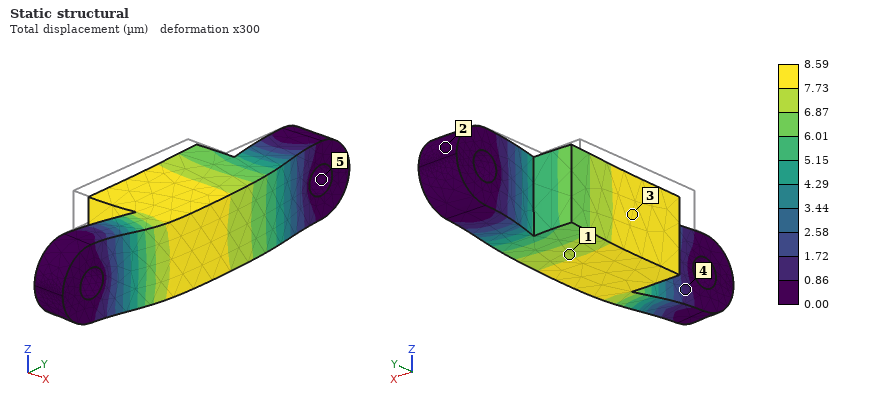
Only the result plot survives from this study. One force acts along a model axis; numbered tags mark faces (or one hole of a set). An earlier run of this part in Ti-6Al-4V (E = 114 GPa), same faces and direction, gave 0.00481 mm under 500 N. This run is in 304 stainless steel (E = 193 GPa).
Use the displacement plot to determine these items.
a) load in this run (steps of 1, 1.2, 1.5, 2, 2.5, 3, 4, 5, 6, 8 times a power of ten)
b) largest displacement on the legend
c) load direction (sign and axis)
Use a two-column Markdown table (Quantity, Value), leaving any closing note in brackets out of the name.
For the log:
| Quantity | Value |
|---|---|
| load in this run | 1.5 kN |
| largest displacement on the legend | 8.59 µm |
| load direction | +X |
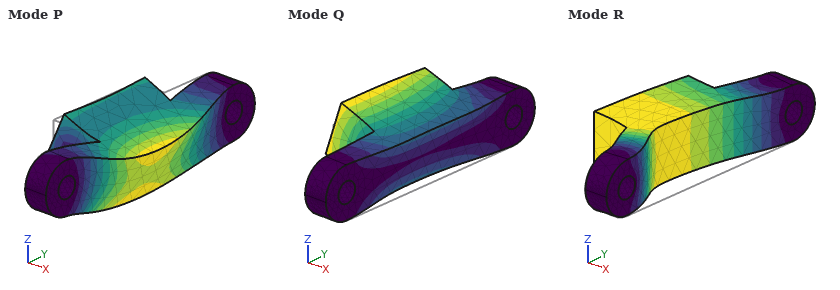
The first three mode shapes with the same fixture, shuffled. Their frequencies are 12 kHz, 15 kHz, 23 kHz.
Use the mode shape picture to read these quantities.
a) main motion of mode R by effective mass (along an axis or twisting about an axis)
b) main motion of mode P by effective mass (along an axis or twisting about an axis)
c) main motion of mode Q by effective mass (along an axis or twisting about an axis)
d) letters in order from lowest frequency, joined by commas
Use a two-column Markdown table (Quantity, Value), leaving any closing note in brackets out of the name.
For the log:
| Quantity | Value |
|---|---|
| main motion of mode R by effective mass | along X |
| main motion of mode P by effective mass | along Z |
| main motion of mode Q by effective mass | along Z |
| letters in order from lowest frequency, joined by commas | Q, R, P |
